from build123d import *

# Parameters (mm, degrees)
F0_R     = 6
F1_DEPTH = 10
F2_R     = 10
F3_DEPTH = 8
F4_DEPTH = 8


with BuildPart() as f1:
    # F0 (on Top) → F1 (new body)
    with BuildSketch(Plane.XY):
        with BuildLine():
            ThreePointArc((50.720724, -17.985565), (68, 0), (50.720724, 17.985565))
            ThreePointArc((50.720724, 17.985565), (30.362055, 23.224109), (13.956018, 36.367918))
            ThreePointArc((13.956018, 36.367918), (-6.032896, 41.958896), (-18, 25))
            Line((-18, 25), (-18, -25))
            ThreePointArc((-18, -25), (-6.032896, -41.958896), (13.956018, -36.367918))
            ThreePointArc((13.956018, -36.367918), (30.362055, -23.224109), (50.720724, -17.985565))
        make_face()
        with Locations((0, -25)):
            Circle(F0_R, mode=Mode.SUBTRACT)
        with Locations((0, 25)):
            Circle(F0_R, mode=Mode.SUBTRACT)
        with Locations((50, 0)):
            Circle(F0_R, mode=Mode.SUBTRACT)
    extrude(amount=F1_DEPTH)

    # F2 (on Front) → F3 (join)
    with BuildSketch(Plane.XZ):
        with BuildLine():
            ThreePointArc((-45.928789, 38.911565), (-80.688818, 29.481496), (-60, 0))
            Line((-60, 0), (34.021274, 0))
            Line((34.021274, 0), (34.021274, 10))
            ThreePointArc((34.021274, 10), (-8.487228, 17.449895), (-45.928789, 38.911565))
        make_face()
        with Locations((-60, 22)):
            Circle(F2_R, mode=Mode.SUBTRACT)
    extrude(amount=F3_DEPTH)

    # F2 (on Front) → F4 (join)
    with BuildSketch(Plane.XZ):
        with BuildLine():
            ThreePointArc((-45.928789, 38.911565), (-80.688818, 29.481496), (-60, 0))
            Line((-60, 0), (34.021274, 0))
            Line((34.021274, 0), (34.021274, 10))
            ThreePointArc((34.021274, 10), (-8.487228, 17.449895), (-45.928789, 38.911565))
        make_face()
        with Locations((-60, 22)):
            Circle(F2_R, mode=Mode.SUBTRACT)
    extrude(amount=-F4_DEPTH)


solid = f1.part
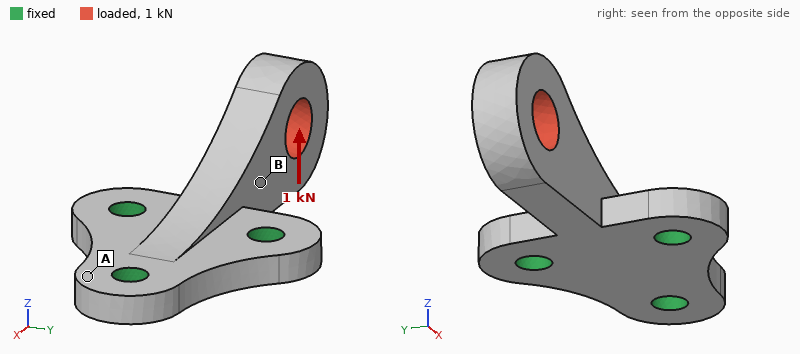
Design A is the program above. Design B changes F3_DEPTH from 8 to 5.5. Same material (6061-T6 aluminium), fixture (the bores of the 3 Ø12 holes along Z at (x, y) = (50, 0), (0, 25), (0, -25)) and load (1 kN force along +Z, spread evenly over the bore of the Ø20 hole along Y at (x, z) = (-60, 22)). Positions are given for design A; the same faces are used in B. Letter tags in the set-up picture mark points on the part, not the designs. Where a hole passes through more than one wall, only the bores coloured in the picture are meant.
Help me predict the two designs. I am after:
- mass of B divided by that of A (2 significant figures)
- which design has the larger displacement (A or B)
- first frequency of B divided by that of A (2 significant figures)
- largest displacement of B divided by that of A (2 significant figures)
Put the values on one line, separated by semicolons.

0.93; B; 1.0; 1.1
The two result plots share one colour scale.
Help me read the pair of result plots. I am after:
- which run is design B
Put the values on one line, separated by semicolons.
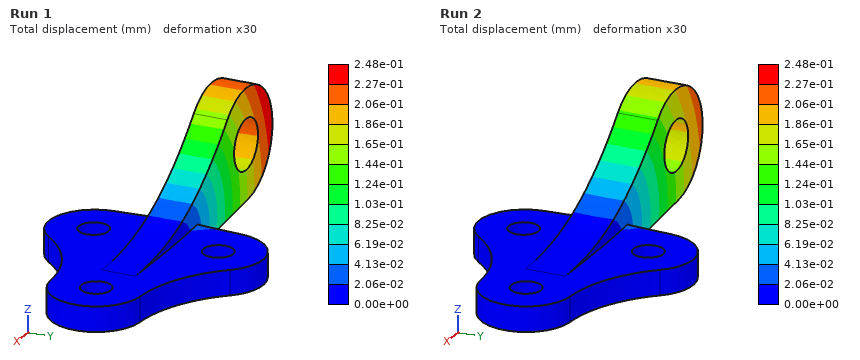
Run 1
